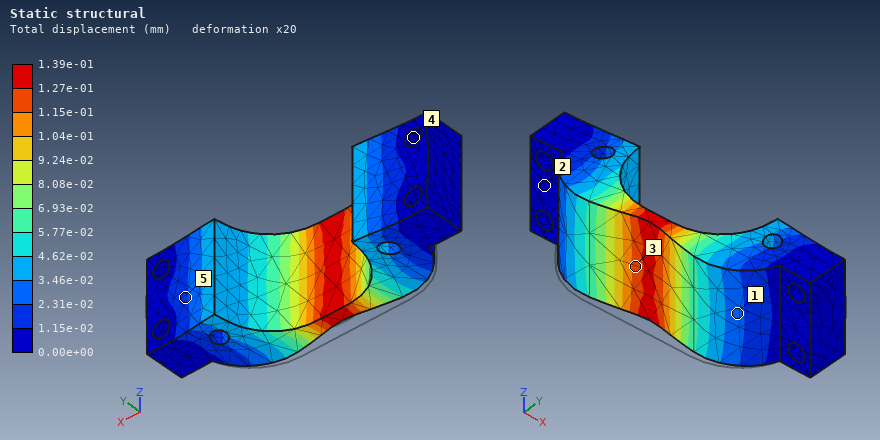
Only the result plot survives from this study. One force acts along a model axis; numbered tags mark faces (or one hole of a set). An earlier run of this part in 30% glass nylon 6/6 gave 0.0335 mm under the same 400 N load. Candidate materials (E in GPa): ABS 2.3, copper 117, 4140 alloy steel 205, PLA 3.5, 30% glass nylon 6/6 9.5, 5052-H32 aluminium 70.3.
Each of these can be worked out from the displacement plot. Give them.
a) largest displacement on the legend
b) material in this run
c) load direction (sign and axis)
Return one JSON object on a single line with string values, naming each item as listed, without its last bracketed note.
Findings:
{"largest displacement on the legend": "1.39e-01 mm", "material in this run": "ABS", "load direction": "+Y"}
